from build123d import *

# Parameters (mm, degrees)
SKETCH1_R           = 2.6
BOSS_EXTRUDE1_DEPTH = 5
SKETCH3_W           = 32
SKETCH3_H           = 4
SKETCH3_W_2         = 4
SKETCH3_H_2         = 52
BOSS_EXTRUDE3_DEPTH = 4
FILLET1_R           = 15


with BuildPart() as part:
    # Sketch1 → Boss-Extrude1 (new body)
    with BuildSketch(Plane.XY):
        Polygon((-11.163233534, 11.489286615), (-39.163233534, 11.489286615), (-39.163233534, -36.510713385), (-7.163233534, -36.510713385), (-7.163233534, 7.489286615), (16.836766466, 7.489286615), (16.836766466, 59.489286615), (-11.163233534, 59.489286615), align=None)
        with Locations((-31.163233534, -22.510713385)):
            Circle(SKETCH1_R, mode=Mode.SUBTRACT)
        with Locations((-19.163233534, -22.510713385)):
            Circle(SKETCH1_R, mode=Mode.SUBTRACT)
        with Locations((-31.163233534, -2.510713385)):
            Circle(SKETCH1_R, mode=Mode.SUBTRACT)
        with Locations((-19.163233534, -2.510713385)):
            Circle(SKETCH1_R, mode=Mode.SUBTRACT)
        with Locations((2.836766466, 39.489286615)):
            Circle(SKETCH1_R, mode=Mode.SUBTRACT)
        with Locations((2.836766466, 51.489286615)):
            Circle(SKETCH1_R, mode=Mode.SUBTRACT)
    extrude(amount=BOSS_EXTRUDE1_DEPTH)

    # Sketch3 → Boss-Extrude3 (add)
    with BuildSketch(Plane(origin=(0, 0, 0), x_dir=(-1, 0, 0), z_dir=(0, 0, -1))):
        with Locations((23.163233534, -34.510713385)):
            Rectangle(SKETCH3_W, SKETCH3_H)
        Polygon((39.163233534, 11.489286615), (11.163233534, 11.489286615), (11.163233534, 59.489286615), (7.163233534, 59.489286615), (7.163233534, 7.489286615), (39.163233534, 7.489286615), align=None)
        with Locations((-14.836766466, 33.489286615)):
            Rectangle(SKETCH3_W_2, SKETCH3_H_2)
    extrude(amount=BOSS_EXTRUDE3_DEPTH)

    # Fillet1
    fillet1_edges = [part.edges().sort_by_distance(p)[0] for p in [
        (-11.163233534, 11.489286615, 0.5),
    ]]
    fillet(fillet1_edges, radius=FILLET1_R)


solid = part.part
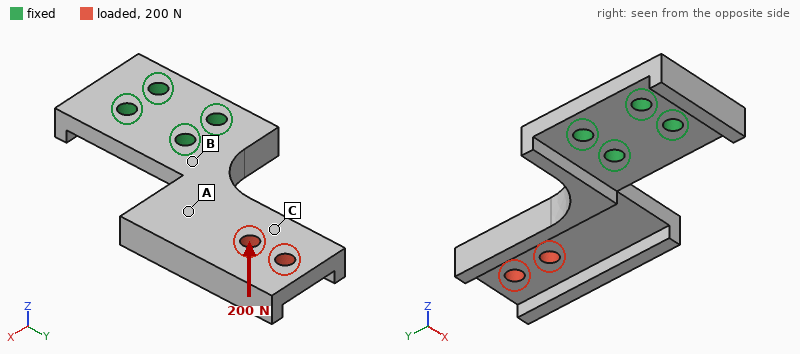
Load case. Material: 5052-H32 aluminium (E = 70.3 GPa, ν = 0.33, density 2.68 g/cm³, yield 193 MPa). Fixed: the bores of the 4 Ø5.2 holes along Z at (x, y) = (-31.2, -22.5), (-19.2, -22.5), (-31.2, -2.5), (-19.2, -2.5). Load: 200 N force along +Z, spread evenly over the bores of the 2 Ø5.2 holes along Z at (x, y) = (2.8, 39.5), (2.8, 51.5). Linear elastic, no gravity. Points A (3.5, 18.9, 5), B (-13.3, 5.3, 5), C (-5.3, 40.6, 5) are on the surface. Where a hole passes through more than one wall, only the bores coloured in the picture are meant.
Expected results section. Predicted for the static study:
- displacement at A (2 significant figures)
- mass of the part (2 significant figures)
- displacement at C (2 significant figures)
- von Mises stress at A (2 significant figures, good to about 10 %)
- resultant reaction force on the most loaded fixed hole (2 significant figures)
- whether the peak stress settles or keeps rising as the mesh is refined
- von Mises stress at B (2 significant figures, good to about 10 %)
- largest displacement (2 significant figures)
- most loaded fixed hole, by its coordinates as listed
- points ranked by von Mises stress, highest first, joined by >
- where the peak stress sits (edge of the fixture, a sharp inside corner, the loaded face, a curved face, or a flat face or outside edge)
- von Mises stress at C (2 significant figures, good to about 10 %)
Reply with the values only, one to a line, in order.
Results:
0.16 mm
46 g
0.32 mm
19 MPa
460 N
keeps rising
85 MPa
0.60 mm
(-19.2, -2.5)
B > A > C
edge of the fixture
8.5 MPa
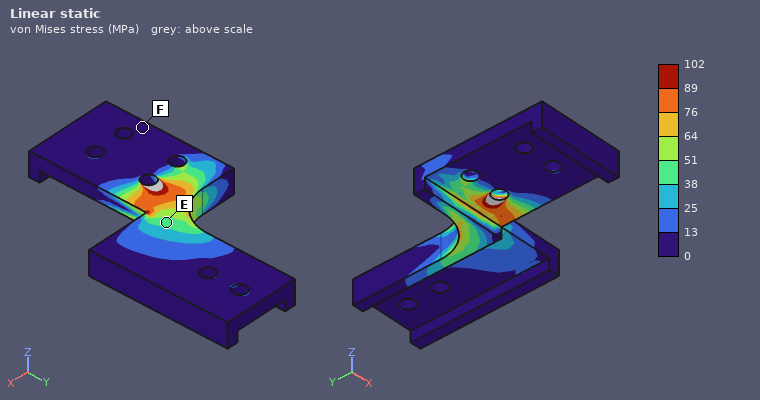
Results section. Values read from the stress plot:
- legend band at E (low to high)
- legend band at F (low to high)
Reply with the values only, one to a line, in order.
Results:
38 to 51 MPa
0 to 13 MPa
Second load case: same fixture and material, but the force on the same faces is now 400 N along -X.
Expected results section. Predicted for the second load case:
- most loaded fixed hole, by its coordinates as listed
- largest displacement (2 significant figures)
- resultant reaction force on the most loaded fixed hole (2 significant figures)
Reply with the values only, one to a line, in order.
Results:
(-31.2, -2.5)
0.21 mm
990 N
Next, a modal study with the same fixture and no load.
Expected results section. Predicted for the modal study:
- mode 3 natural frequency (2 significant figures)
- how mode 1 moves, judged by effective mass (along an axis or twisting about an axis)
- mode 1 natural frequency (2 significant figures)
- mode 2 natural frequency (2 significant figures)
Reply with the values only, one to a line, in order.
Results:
2900 Hz
along Z
910 Hz
2100 Hz
